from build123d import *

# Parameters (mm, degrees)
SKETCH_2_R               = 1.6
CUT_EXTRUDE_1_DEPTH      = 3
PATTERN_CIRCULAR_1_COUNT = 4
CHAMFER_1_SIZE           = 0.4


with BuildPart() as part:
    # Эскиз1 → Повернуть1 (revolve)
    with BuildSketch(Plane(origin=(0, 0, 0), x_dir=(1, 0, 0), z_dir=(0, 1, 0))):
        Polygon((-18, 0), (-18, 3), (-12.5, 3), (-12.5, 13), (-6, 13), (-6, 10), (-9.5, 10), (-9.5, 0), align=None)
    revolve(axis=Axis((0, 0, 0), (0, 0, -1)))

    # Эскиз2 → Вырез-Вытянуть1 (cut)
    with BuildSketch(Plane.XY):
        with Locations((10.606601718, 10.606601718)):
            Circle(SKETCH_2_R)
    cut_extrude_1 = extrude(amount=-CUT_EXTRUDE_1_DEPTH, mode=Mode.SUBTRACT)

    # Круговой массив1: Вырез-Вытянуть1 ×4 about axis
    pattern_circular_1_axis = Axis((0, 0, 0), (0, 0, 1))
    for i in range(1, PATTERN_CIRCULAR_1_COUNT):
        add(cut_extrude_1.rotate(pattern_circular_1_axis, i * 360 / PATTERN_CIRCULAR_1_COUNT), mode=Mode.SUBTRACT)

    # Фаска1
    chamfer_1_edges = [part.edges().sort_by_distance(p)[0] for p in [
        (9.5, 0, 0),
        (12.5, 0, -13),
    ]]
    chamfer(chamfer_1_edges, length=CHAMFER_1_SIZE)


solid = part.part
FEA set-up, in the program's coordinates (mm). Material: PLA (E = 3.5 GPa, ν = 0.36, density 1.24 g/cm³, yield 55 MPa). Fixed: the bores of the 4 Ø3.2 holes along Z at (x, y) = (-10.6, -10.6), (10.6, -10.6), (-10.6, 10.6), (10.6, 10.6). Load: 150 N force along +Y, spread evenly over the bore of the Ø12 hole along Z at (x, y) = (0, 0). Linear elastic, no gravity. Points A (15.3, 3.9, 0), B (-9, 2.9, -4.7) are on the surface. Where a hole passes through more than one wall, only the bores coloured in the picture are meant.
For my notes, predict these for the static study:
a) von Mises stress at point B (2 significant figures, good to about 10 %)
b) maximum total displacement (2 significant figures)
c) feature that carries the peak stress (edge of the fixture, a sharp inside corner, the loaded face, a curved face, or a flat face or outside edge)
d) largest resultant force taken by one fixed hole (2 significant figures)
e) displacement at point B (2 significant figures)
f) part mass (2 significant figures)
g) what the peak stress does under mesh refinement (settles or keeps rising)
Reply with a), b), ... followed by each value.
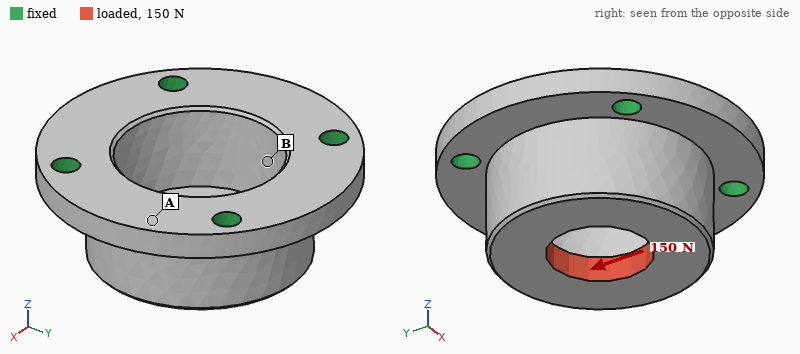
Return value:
a) 2.5 MPa
b) 26 µm
c) edge of the fixture
d) 53 N
e) 5.1 µm
f) 5.8 g
g) keeps rising
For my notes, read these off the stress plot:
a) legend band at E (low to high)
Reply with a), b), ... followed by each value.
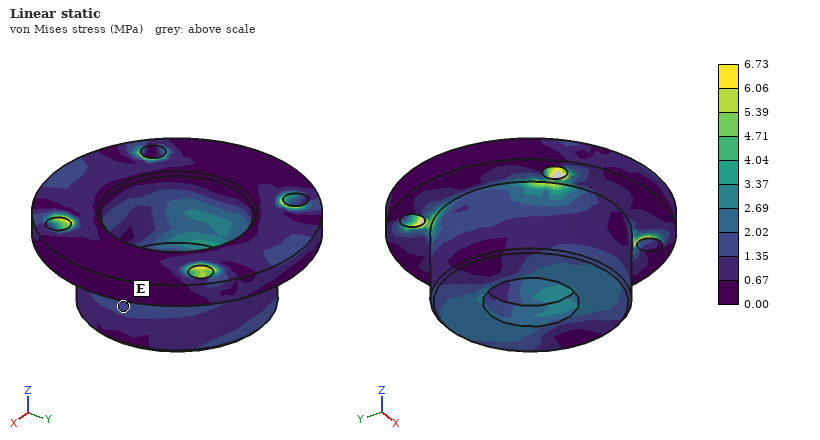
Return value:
a) 1.35 to 2.02 MPa
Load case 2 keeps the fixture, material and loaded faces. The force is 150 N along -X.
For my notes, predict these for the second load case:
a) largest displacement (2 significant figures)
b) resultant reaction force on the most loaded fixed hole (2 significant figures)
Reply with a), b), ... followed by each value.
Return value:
a) 26 µm
b) 53 N
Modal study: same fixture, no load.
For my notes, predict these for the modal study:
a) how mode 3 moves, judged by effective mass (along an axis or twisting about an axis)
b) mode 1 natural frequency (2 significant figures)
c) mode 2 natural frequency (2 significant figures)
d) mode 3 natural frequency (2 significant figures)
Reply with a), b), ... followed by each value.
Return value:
a) along Z
b) 9000 Hz
c) 9000 Hz
d) 11 kHz
